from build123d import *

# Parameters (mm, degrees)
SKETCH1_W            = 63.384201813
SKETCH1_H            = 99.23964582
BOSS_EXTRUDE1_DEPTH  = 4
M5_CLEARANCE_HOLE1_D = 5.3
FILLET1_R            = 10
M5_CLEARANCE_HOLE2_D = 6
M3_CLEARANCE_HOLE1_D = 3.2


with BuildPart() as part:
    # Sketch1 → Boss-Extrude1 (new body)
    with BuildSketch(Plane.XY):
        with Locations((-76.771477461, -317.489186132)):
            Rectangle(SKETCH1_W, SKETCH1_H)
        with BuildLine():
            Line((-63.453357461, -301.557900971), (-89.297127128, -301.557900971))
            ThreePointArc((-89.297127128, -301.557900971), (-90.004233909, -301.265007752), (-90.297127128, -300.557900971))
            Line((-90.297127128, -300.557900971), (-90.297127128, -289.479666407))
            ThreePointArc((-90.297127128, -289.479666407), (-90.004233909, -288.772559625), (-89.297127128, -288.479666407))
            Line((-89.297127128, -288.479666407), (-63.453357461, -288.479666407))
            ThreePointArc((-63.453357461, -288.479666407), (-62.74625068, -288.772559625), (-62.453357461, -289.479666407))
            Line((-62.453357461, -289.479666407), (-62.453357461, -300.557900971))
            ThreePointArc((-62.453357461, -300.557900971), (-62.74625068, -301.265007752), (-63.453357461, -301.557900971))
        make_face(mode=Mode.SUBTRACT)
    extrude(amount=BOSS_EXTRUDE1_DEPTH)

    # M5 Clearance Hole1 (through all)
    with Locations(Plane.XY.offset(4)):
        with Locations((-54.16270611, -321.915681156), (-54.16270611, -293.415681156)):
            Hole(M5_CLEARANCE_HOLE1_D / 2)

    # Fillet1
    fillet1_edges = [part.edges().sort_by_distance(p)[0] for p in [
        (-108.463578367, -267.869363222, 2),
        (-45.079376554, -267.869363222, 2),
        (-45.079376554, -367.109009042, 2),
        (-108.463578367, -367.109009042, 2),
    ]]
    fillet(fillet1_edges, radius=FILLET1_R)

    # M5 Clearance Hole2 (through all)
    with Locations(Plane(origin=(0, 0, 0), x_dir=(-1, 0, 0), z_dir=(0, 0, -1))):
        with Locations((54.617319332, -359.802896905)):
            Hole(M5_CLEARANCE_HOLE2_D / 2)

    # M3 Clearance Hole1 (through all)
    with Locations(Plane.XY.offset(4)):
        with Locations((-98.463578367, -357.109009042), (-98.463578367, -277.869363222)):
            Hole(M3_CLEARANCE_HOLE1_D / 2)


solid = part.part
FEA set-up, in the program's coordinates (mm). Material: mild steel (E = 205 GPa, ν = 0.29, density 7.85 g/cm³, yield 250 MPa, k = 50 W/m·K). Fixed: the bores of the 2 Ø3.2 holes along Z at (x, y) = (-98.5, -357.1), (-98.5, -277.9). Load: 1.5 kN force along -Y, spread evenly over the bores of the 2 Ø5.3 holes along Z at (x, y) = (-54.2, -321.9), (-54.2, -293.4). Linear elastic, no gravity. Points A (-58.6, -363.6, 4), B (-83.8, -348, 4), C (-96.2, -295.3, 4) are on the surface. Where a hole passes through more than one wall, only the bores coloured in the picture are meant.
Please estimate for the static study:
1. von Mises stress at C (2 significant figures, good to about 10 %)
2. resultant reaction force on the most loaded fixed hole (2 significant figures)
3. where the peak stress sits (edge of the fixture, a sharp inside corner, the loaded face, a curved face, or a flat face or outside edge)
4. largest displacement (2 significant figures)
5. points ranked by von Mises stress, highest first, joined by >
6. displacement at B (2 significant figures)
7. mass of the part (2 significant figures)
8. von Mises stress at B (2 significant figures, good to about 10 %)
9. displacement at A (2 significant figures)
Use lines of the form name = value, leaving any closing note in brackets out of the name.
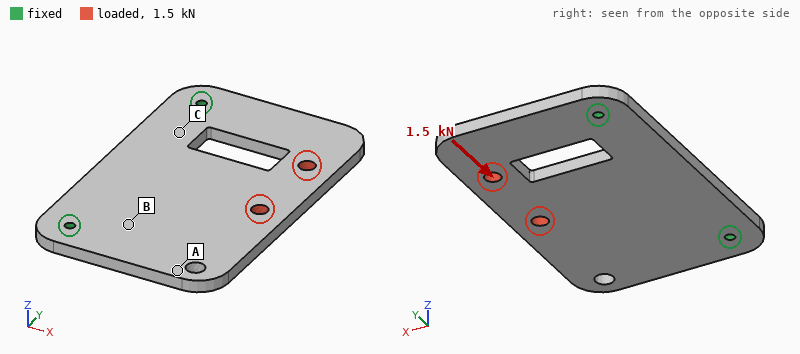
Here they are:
von Mises stress at C = 17 MPa
resultant reaction force on the most loaded fixed hole = 1.2 kN
where the peak stress sits = a curved face
largest displacement = 7.4 µm
points ranked by von Mises stress, highest first, joined by > = C > B > A
displacement at B = 2.2 µm
mass of the part = 180 g
von Mises stress at B = 10 MPa
displacement at A = 5.6 µm
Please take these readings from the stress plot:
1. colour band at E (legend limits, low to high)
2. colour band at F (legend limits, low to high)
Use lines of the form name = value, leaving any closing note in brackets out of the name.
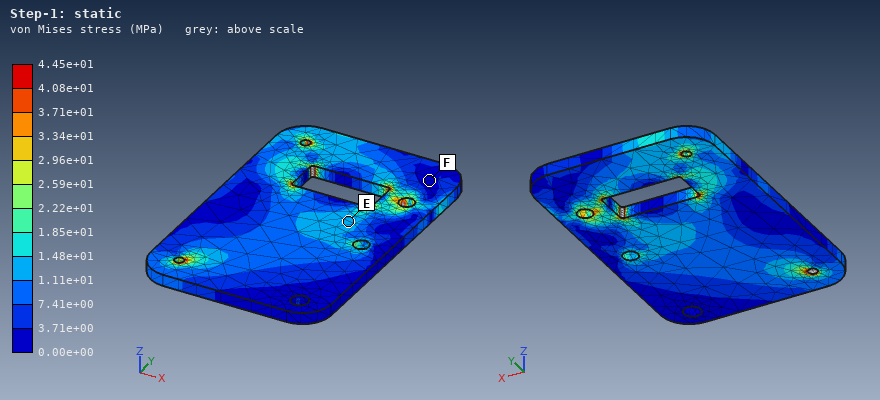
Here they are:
colour band at E = 1.11e+01 to 1.48e+01 MPa
colour band at F = 0.00e+00 to 3.71e+00 MPa
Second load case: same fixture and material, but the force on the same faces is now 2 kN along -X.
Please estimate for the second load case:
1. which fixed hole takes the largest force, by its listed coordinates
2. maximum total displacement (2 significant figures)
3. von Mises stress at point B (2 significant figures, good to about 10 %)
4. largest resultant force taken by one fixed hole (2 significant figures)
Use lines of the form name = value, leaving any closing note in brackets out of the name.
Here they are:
which fixed hole takes the largest force, by its listed coordinates = (-98.5, -277.9)
maximum total displacement = 6.2 µm
von Mises stress at point B = 8.9 MPa
largest resultant force taken by one fixed hole = 1.3 kN
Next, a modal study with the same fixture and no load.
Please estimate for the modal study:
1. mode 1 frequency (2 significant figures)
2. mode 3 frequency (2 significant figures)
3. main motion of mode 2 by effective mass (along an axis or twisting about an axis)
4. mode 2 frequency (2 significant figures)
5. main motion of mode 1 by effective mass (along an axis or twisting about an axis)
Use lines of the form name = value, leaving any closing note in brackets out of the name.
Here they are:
mode 1 frequency = 850 Hz
mode 3 frequency = 2800 Hz
main motion of mode 2 by effective mass = twisting about X
mode 2 frequency = 1800 Hz
main motion of mode 1 by effective mass = along Z
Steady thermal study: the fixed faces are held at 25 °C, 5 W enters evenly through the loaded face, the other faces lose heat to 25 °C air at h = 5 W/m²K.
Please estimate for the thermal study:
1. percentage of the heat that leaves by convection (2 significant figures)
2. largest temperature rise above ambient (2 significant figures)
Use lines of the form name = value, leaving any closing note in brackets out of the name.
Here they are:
percentage of the heat that leaves by convection = 13 %
largest temperature rise above ambient = 22 K
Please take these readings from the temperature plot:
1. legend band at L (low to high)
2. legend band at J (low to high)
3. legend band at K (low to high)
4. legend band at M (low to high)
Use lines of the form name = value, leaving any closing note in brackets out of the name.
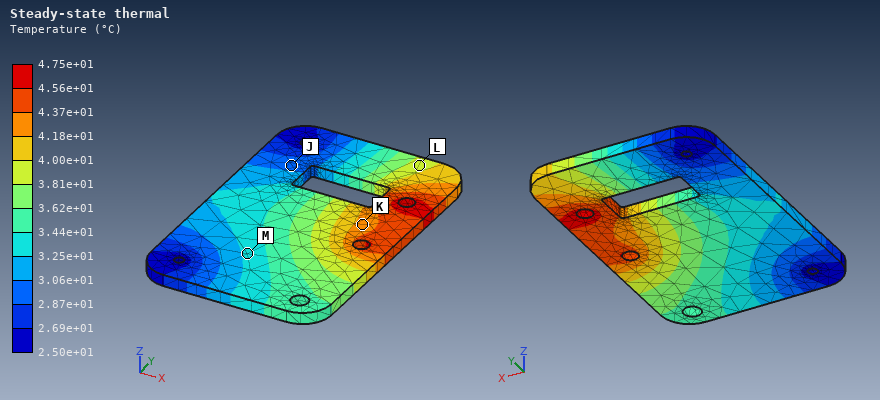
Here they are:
legend band at L = 3.81e+01 to 4.00e+01 °C
legend band at J = 2.87e+01 to 3.06e+01 °C
legend band at K = 4.18e+01 to 4.37e+01 °C
legend band at M = 3.25e+01 to 3.44e+01 °C
